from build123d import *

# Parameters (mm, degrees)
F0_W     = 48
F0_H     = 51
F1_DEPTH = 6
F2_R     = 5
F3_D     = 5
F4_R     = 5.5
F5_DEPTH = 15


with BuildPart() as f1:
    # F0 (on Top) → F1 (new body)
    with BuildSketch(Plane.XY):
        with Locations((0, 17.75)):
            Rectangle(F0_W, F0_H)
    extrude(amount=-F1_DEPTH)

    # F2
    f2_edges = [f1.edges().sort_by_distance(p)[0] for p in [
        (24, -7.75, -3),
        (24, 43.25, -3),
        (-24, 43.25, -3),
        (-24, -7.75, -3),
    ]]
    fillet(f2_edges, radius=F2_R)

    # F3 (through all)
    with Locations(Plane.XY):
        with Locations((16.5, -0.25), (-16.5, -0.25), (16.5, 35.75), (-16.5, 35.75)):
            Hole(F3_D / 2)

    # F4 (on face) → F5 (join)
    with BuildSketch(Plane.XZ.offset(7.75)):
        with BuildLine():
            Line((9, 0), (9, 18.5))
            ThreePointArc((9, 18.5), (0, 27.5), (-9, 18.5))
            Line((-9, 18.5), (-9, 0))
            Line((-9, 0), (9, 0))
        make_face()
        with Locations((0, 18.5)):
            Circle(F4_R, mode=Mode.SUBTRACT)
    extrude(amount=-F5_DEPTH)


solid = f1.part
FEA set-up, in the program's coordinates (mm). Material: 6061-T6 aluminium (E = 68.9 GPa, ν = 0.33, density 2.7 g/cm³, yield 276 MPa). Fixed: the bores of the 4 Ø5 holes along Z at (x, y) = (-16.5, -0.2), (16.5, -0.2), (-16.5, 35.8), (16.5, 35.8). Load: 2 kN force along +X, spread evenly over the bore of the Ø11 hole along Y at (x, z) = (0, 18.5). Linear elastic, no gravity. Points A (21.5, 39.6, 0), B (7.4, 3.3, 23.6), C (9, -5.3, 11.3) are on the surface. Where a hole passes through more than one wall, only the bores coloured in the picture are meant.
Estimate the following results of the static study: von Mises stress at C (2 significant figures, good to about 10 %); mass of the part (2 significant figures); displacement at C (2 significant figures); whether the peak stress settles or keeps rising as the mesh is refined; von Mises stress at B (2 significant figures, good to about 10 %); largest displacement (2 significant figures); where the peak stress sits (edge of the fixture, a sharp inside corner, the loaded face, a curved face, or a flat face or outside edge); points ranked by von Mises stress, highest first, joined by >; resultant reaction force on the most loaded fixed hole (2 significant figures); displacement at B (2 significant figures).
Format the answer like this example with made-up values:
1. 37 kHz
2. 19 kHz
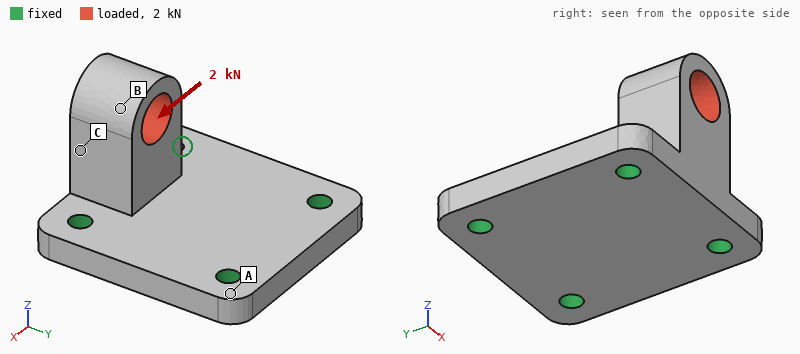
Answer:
1. 37 MPa
2. 53 g
3. 26 µm
4. keeps rising
5. 25 MPa
6. 64 µm
7. edge of the fixture
8. C > B > A
9. 1.9 kN
10. 60 µm
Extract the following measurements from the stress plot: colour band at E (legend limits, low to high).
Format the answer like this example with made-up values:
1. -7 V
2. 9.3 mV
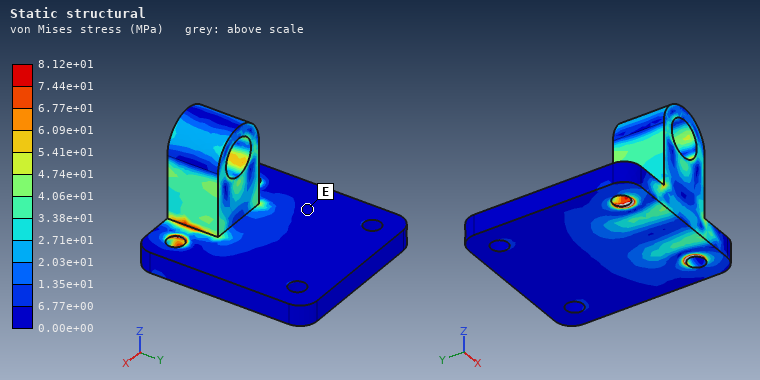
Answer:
1. 0.00e+00 to 6.77e+00 MPa
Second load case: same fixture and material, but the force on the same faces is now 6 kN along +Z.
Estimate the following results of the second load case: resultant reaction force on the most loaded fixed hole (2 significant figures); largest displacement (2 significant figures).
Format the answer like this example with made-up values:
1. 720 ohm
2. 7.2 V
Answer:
1. 3.1 kN
2. 52 µm
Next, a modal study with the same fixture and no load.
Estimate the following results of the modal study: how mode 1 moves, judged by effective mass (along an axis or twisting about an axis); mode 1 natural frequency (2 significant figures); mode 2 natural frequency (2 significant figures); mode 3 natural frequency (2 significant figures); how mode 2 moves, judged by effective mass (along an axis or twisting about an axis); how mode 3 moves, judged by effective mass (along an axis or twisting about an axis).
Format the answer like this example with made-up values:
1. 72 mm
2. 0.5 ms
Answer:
1. along Y
2. 7500 Hz
3. 12 kHz
4. 16 kHz
5. along X
6. along Z
